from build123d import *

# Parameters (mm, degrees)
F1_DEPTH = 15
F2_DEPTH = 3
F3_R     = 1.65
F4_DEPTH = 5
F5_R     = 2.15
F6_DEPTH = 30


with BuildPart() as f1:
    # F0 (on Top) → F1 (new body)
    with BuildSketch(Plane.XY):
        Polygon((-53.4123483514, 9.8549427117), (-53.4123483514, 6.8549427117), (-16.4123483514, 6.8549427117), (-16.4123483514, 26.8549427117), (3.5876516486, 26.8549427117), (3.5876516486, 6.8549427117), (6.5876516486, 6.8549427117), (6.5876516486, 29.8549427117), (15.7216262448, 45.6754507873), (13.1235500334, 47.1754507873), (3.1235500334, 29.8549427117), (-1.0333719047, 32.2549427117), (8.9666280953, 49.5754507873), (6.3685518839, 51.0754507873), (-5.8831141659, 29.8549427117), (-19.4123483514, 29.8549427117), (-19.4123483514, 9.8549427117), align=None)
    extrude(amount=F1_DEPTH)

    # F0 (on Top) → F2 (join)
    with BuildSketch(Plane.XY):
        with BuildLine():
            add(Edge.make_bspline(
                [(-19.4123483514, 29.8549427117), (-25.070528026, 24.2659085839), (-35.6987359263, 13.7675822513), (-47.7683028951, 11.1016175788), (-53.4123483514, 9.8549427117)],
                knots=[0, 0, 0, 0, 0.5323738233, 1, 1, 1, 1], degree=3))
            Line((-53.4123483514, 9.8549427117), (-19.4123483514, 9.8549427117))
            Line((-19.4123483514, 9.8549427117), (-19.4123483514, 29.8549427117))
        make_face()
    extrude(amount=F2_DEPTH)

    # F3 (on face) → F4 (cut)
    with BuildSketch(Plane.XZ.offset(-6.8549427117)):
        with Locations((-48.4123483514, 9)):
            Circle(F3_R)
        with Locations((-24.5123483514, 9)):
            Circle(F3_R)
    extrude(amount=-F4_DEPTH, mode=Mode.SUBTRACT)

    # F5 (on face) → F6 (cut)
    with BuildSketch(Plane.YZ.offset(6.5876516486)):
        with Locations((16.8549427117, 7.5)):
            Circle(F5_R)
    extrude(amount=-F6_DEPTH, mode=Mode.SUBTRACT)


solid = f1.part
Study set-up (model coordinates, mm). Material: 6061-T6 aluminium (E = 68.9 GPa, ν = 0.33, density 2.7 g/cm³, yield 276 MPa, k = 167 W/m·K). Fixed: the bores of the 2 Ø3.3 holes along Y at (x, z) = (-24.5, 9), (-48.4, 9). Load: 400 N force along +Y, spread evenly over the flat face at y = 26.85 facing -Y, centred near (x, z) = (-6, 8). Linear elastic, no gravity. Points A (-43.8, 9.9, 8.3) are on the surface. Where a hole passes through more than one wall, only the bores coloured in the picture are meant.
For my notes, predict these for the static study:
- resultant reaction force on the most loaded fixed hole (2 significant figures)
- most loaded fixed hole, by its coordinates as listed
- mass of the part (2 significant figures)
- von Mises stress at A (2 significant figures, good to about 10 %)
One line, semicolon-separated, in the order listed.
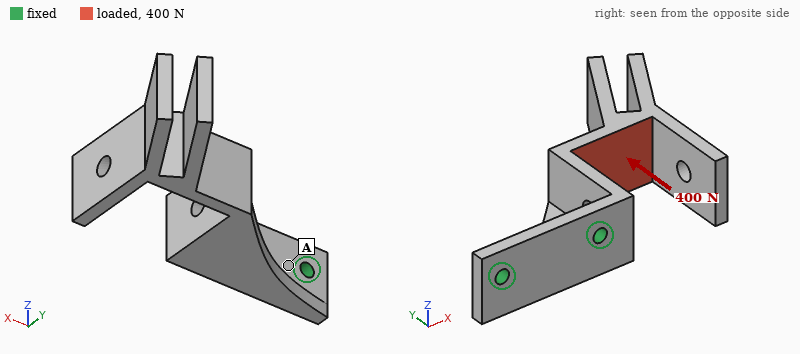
640 N; (-24.5, 9); 19 g; 23 MPa
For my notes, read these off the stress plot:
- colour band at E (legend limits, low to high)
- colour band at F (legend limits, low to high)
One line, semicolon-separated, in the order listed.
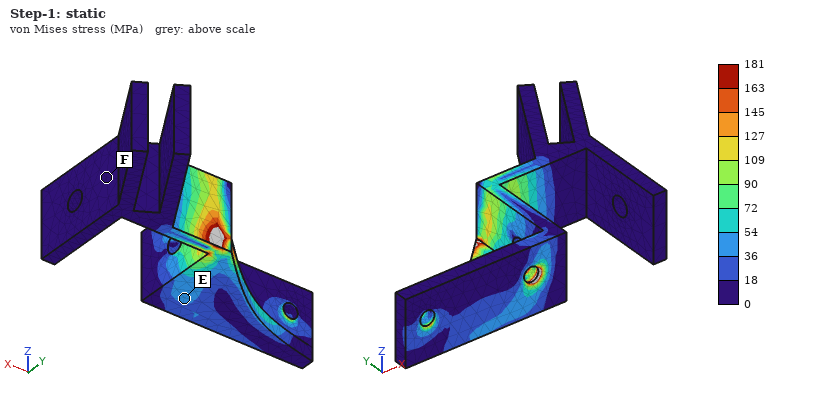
36 to 54 MPa; 0 to 18 MPa
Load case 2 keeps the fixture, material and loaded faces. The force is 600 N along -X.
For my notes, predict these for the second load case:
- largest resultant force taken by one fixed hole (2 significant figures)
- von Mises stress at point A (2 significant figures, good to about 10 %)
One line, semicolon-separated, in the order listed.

500 N; 47 MPa
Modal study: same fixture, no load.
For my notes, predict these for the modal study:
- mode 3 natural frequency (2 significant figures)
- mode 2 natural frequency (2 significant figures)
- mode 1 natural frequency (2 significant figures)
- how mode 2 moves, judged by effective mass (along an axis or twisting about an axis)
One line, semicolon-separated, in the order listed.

2200 Hz; 1200 Hz; 780 Hz; along Z
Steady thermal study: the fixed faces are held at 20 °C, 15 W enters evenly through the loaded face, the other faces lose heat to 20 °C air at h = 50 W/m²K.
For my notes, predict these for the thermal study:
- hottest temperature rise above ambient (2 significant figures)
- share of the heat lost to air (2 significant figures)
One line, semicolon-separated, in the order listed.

35 K; 37 %
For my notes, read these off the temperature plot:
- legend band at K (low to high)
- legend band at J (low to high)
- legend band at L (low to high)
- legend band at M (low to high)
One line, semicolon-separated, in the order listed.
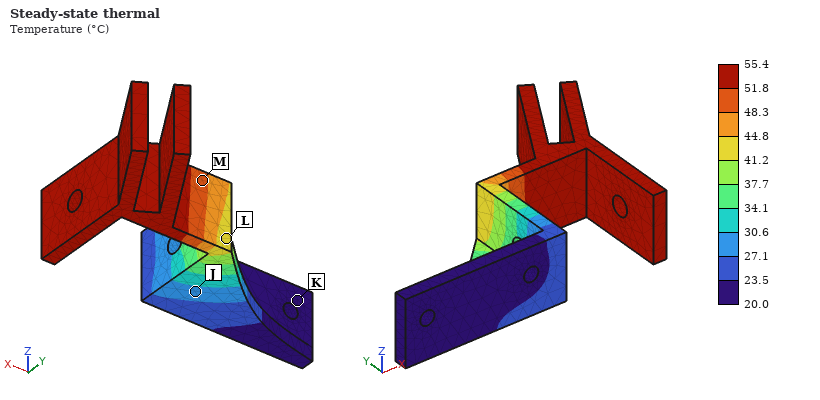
20.0 to 23.5 °C; 27.1 to 30.6 °C; 41.2 to 44.8 °C; 48.3 to 51.8 °C
